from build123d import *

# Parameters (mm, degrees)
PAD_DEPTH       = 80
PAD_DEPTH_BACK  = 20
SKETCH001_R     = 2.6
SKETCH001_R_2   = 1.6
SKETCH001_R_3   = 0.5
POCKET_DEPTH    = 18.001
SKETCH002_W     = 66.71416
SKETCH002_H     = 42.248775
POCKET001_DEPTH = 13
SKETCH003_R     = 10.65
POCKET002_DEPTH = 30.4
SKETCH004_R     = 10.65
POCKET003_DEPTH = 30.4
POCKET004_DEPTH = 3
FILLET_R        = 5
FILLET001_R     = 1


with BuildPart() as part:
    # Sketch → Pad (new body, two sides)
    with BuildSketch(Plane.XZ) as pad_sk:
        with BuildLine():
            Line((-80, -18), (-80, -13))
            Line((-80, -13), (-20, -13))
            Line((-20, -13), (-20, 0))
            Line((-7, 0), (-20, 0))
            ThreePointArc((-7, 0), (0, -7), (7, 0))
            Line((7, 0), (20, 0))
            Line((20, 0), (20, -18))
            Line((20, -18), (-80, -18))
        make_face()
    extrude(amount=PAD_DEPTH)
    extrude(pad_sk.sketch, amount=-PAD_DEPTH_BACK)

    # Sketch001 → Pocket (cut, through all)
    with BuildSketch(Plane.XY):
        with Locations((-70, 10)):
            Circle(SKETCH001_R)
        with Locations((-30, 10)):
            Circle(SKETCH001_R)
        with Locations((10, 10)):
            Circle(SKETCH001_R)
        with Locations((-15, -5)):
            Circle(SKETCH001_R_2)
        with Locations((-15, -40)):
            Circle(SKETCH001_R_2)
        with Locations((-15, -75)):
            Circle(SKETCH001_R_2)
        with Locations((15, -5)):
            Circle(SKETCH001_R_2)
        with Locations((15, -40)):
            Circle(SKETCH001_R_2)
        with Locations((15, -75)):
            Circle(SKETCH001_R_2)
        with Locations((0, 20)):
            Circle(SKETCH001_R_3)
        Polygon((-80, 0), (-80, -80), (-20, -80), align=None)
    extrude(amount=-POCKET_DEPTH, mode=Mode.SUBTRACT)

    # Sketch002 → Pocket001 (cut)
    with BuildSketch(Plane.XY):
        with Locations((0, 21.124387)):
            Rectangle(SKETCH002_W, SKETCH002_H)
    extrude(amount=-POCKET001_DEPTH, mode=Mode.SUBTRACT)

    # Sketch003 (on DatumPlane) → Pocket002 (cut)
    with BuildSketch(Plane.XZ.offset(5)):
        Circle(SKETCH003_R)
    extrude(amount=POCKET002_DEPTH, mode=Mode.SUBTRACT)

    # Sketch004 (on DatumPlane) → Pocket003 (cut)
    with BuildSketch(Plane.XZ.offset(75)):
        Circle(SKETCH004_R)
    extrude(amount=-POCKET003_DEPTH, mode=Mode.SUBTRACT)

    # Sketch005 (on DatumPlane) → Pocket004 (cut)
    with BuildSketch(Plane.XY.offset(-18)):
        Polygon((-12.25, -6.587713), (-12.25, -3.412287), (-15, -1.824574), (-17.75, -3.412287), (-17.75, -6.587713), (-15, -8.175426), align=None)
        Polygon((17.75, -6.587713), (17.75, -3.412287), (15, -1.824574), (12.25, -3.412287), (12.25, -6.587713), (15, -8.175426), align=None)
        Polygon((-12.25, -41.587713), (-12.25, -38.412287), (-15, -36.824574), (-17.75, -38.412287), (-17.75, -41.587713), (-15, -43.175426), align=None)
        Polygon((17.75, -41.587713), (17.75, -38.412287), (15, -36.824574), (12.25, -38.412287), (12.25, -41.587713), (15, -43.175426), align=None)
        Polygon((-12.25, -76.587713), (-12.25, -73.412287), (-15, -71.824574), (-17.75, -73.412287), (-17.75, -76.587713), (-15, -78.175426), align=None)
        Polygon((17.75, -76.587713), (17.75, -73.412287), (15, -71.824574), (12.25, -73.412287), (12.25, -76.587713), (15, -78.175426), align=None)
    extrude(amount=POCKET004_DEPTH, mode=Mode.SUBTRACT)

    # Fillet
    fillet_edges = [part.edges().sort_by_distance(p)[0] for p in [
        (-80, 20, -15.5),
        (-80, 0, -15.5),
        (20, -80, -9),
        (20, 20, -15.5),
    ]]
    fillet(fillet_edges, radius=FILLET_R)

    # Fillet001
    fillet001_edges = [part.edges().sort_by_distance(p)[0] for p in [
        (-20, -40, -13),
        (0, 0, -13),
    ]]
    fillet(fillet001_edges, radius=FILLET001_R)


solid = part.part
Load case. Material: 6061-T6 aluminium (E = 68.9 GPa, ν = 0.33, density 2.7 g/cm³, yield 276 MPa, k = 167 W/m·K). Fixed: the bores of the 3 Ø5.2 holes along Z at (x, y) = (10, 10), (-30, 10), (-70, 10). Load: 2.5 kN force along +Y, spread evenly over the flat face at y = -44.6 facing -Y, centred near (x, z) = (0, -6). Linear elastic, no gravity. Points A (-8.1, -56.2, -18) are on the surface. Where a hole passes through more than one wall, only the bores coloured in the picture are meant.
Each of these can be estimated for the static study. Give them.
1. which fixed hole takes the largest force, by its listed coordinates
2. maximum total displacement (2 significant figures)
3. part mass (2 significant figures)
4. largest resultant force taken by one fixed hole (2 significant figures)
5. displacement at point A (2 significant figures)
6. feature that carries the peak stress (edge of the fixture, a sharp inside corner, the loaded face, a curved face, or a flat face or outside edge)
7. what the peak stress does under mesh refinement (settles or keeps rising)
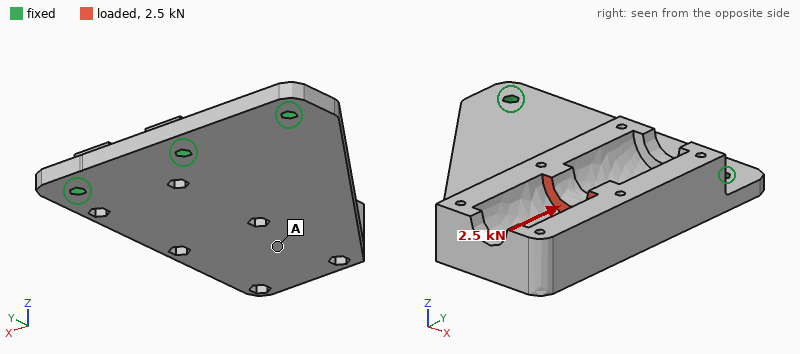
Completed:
(10, 10)
0.61 mm
180 g
1.7 kN
0.41 mm
edge of the fixture
keeps rising
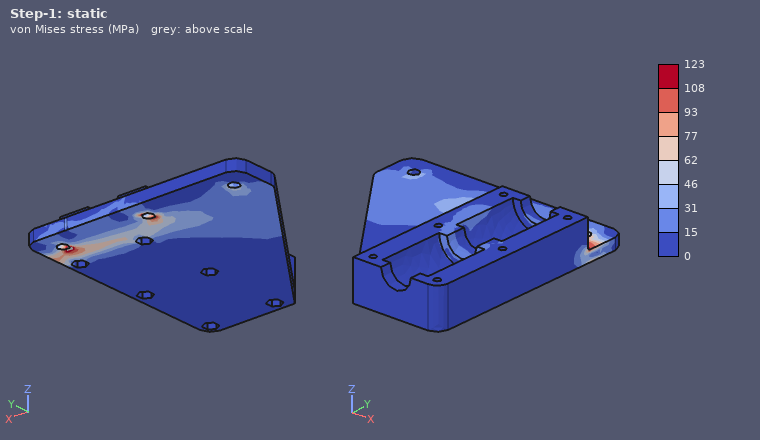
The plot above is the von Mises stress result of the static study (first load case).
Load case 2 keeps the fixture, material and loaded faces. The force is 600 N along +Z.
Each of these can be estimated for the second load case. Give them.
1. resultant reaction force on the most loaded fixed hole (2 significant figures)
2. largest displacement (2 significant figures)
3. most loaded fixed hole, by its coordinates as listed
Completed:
460 N
0.73 mm
(10, 10)
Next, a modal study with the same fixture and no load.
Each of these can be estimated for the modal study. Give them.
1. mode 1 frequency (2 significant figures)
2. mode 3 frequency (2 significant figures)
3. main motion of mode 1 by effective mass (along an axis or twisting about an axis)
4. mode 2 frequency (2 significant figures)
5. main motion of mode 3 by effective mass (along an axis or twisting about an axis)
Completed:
520 Hz
4700 Hz
along Z
2700 Hz
along X
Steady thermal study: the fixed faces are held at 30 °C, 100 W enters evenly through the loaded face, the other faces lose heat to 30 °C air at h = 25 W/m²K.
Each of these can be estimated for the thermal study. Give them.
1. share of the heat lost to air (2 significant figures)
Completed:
18 %
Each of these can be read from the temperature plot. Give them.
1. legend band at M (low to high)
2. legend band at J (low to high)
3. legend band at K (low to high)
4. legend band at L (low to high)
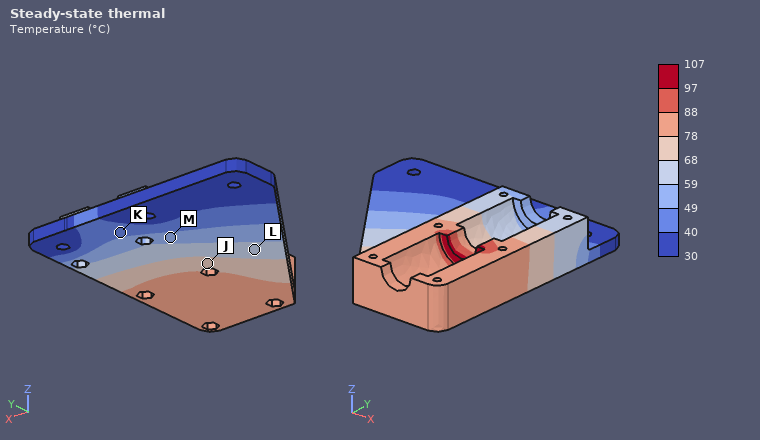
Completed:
49 to 59 °C
68 to 78 °C
40 to 49 °C
59 to 68 °C
